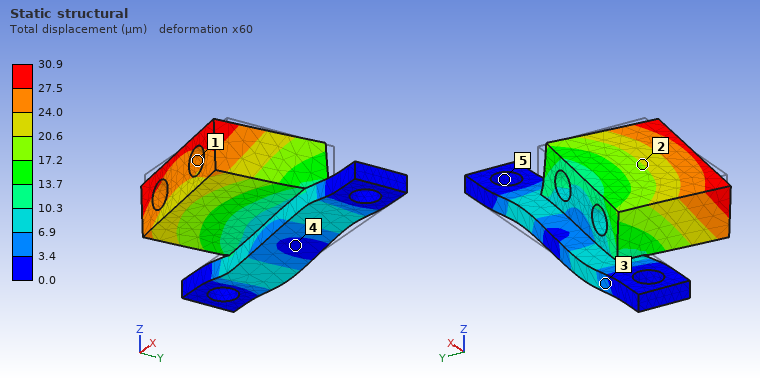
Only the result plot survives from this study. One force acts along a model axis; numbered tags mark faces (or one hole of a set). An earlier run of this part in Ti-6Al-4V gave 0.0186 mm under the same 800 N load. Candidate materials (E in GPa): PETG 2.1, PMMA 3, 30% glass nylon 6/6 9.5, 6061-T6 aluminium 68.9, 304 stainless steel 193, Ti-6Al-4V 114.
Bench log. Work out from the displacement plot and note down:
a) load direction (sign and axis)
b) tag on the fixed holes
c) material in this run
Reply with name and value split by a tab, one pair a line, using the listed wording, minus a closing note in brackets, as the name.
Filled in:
load direction	-X
tag on the fixed holes	5
material in this run	6061-T6 aluminium
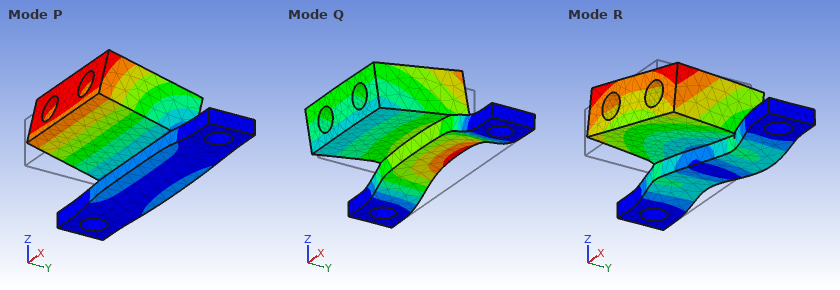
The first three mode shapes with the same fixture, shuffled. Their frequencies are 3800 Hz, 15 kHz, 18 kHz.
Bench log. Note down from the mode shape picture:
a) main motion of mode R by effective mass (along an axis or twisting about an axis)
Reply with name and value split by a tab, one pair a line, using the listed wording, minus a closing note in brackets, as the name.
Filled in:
main motion of mode R by effective mass	along X
